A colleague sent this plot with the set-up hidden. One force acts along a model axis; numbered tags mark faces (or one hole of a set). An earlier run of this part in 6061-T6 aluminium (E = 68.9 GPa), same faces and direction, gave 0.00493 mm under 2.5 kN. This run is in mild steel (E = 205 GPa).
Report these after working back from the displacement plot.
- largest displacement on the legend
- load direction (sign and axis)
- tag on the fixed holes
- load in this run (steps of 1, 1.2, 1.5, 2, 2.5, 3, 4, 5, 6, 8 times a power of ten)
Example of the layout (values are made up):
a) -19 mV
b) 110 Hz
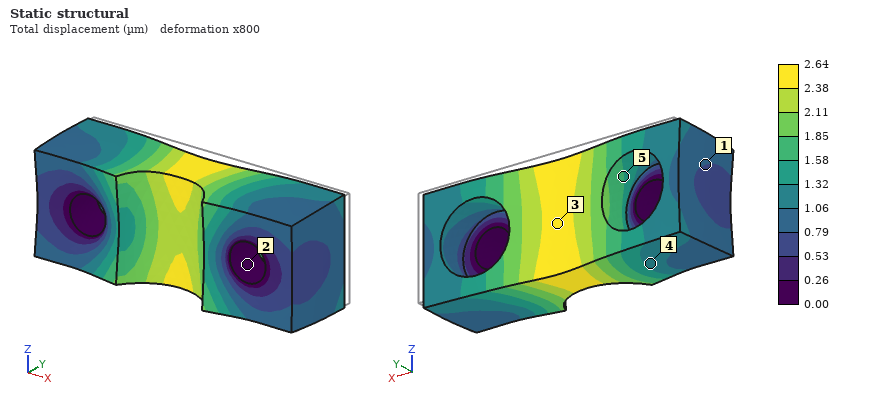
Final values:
a) 2.64 µm
b) -Y
c) 2
d) 4 kN
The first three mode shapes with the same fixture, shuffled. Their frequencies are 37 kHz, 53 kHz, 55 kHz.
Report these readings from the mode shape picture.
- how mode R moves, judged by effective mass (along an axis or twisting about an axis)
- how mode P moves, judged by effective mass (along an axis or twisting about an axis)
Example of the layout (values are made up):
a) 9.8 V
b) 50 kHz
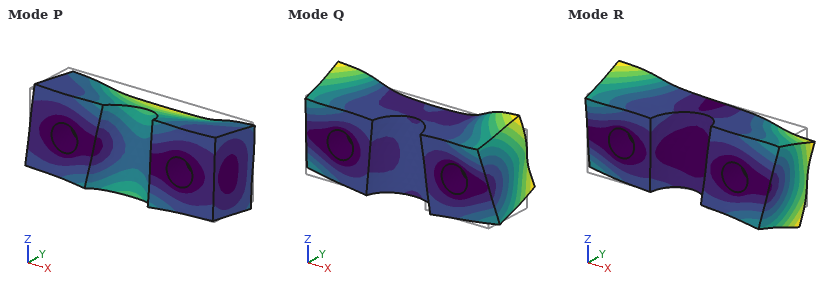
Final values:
a) twisting about Y
b) along Z
